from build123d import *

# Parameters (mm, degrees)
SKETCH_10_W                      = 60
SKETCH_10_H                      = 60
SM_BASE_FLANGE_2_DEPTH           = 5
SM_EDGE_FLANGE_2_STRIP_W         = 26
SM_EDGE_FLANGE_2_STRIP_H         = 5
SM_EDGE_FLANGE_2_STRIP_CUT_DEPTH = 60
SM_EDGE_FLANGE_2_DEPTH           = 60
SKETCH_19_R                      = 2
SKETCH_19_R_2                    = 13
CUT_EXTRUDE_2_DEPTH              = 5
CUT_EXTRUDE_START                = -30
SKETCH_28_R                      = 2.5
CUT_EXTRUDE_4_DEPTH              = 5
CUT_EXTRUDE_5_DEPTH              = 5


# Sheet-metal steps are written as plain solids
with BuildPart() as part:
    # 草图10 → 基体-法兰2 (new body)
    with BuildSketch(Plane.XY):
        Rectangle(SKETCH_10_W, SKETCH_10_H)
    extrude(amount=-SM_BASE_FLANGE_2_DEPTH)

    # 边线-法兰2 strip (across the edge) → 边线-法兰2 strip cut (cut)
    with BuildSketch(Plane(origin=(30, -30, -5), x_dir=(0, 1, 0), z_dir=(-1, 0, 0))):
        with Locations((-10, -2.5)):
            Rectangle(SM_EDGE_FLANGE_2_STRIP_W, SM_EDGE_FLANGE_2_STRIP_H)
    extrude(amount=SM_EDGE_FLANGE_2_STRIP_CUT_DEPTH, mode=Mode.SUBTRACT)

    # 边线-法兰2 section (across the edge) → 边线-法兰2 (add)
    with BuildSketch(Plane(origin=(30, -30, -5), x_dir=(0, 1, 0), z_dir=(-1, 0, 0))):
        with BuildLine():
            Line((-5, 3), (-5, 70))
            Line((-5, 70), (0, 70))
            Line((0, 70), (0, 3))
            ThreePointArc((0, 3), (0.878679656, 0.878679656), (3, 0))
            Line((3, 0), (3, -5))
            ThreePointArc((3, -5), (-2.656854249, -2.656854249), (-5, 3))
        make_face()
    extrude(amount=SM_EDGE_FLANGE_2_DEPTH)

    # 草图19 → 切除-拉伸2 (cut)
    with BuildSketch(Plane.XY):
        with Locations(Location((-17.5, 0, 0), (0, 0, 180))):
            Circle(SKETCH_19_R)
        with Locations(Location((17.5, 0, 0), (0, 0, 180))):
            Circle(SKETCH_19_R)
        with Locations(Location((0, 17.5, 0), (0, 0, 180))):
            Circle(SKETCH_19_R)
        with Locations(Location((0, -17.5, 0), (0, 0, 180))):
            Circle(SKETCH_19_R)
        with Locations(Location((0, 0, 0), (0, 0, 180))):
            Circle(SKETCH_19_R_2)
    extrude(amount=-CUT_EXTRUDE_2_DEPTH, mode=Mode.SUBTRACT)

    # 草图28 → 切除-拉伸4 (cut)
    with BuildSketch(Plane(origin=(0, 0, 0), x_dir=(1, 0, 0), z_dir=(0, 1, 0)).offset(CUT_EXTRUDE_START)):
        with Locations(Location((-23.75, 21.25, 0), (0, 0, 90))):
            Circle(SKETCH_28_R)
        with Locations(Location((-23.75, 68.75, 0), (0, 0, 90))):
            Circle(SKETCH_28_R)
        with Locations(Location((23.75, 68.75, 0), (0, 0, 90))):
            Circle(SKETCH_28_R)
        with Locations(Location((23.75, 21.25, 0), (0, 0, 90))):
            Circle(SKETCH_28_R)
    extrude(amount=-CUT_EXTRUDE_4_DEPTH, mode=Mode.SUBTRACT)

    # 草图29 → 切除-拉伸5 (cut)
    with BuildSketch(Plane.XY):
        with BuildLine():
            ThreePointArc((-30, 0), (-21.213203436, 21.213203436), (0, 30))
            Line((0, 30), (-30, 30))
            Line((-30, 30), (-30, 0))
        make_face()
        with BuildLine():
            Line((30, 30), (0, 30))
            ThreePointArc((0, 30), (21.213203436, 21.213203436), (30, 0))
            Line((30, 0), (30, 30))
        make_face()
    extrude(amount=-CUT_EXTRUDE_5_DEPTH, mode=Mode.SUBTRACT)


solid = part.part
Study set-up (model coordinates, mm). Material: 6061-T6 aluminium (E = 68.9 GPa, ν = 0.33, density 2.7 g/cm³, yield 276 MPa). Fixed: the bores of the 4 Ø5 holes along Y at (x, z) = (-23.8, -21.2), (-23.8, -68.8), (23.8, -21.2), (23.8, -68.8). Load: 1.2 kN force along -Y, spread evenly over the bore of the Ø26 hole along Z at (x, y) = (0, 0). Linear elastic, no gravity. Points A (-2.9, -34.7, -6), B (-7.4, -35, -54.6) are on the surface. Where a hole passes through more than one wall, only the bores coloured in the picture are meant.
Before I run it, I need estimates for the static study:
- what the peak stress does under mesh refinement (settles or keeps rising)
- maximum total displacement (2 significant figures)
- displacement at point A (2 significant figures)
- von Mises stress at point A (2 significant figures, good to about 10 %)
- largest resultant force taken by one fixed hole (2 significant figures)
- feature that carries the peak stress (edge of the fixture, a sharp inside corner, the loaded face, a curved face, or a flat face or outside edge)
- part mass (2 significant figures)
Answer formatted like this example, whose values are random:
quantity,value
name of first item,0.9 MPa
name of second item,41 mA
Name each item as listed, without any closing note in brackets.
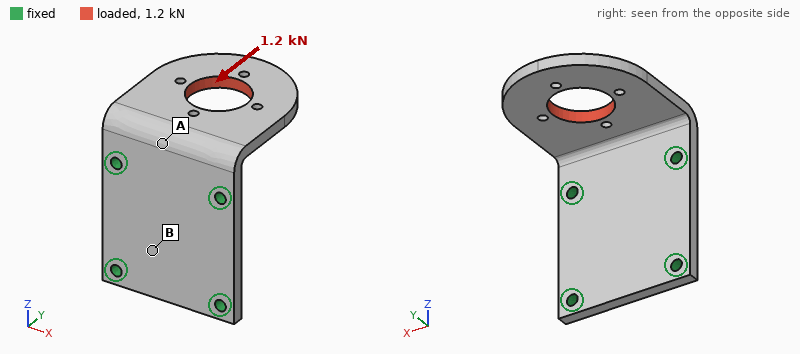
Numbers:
quantity,value
what the peak stress does under mesh refinement,keeps rising
maximum total displacement,0.35 mm
displacement at point A,0.061 mm
von Mises stress at point A,17 MPa
largest resultant force taken by one fixed hole,650 N
feature that carries the peak stress,edge of the fixture
part mass,93 g
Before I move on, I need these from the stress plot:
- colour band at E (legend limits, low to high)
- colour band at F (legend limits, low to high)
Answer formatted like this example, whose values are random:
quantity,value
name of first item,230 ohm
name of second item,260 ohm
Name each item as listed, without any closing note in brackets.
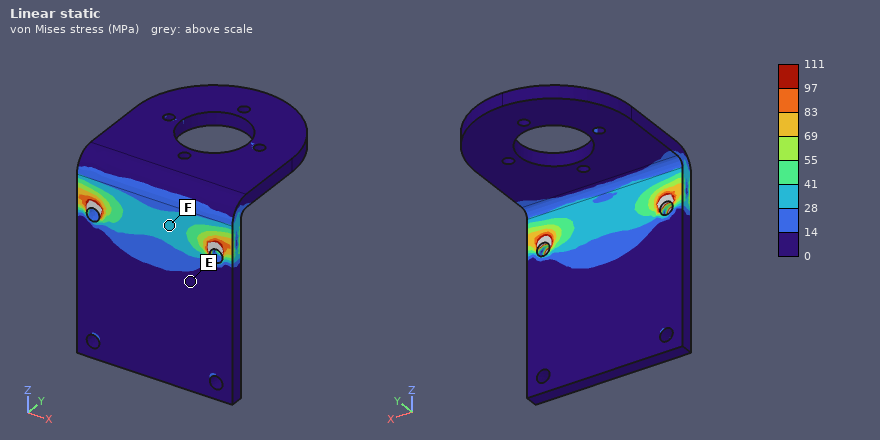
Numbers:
quantity,value
colour band at E,0 to 14 MPa
colour band at F,28 to 41 MPa
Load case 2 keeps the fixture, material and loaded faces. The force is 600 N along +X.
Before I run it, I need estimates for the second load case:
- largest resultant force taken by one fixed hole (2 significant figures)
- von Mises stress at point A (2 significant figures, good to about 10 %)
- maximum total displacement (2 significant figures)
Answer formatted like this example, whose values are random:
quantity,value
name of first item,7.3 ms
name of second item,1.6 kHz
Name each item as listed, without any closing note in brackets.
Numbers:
quantity,value
largest resultant force taken by one fixed hole,560 N
von Mises stress at point A,12 MPa
maximum total displacement,95 µm
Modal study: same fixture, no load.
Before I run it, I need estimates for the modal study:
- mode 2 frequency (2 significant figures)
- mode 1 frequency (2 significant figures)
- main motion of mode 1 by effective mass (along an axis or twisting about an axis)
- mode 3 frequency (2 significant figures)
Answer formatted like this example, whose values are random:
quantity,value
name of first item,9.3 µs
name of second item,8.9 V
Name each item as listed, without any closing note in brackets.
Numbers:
quantity,value
mode 2 frequency,2200 Hz
mode 1 frequency,880 Hz
main motion of mode 1 by effective mass,along Z
mode 3 frequency,3300 Hz
